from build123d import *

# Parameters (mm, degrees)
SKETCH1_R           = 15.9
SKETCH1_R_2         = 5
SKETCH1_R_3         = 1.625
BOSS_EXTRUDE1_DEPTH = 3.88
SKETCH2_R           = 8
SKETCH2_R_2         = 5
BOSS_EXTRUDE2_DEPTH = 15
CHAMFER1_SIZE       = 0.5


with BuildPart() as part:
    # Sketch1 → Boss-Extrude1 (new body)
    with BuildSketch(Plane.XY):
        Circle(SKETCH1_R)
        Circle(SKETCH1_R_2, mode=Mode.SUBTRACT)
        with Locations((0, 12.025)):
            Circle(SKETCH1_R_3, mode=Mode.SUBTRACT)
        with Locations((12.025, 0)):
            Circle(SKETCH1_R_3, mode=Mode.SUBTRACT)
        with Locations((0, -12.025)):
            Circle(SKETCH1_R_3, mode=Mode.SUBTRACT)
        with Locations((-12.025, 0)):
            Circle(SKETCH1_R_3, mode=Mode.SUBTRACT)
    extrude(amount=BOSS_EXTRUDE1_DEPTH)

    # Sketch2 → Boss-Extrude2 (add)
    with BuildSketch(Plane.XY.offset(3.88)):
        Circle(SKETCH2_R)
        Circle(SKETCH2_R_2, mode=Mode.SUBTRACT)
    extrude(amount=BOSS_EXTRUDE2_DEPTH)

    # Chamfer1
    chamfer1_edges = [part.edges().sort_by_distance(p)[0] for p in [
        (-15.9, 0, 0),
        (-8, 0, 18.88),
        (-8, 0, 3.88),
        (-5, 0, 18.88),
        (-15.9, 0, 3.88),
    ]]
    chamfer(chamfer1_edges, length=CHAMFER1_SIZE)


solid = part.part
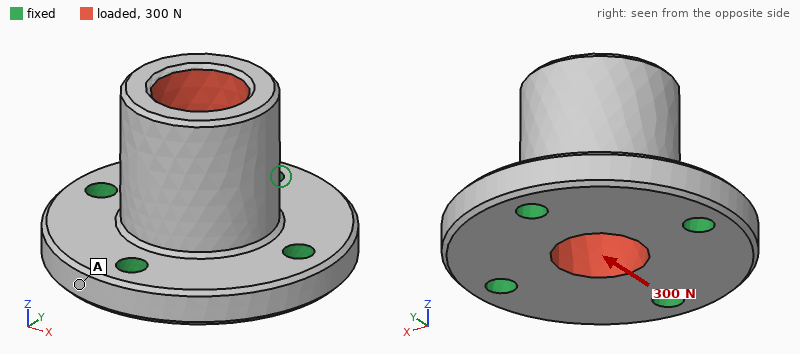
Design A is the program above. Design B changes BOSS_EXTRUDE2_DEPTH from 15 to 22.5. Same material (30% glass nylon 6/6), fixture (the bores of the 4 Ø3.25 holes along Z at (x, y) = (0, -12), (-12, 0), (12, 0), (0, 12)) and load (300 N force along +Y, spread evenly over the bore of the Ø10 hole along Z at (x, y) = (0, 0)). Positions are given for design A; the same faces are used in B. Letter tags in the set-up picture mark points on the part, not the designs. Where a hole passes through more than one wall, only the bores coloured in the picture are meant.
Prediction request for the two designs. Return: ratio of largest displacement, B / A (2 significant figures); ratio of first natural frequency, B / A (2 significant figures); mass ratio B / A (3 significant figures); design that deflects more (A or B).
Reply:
2.2
0.59
1.21
B
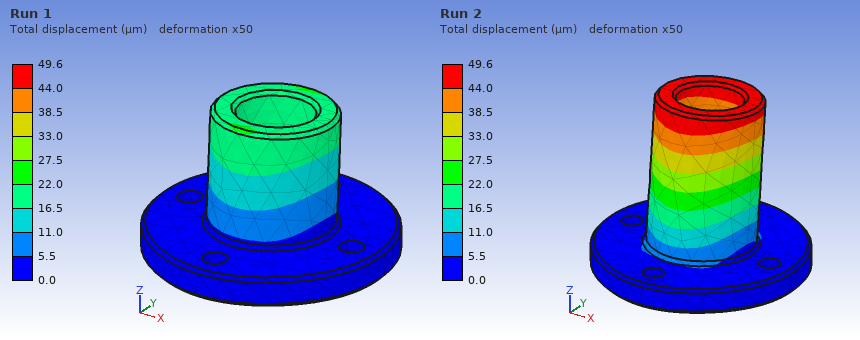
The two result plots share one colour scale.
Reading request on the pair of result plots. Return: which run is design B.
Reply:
Run 2
